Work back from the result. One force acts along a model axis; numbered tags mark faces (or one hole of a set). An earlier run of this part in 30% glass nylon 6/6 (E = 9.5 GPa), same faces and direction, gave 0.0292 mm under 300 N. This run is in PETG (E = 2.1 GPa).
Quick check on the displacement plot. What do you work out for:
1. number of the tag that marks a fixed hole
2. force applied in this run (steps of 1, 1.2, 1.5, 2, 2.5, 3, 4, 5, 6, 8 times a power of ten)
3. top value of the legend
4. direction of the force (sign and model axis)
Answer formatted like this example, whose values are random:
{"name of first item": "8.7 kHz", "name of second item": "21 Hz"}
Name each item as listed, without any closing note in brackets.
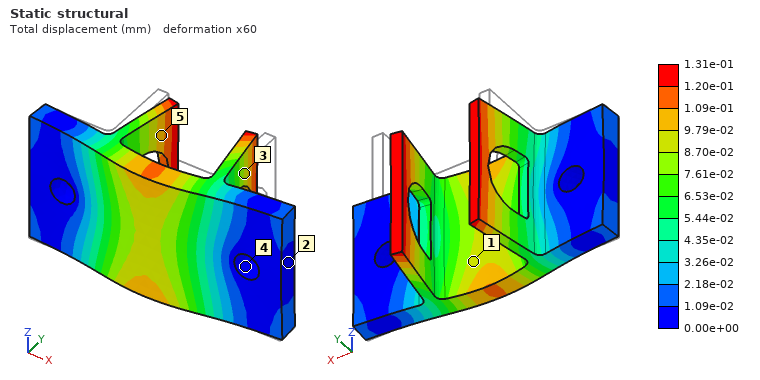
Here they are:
{"number of the tag that marks a fixed hole": "4", "force applied in this run": "300 N", "top value of the legend": "1.31e-01 mm", "direction of the force": "-Y"}
